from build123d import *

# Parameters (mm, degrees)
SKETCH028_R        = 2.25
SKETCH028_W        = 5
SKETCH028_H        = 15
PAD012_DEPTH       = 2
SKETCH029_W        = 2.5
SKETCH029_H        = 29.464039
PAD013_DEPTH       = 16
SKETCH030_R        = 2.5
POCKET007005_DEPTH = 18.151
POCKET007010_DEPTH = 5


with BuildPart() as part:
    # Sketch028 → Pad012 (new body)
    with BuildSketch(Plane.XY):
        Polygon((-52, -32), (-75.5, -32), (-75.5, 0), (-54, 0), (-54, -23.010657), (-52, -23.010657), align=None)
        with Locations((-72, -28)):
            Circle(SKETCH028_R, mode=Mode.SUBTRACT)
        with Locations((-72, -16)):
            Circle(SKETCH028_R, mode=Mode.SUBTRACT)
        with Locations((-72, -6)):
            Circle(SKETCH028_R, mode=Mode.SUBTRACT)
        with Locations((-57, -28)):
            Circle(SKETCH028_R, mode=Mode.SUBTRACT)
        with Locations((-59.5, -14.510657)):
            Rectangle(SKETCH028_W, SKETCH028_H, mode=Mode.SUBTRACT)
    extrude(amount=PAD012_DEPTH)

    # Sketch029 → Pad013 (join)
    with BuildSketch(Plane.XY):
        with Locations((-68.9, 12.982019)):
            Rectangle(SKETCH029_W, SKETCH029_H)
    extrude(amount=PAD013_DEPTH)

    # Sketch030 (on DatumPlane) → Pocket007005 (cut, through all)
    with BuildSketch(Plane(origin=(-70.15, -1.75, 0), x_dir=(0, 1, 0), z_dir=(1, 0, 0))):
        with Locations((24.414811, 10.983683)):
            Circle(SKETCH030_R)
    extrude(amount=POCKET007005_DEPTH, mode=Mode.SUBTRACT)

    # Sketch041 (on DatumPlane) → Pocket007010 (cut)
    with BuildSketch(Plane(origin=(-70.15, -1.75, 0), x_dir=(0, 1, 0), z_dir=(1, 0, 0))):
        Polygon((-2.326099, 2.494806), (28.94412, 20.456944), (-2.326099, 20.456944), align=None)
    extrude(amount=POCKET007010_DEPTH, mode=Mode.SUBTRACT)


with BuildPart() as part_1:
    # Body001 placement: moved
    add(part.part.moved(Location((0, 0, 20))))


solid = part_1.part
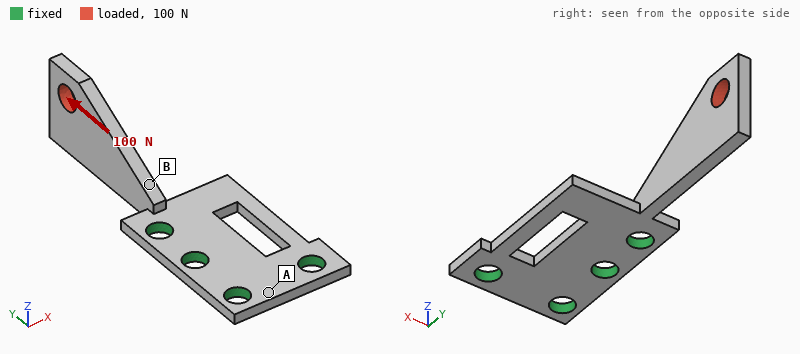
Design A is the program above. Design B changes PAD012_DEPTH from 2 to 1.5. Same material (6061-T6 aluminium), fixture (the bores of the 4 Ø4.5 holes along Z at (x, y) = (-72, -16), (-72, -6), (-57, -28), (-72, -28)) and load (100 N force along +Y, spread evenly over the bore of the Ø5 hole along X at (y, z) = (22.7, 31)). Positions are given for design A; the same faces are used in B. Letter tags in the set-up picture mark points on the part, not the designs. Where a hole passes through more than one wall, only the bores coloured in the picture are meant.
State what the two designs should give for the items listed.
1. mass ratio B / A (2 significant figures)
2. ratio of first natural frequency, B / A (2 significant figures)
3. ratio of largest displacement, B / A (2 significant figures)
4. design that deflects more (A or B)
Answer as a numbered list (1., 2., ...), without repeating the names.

1. 0.85
2. 0.72
3. 1.9
4. B
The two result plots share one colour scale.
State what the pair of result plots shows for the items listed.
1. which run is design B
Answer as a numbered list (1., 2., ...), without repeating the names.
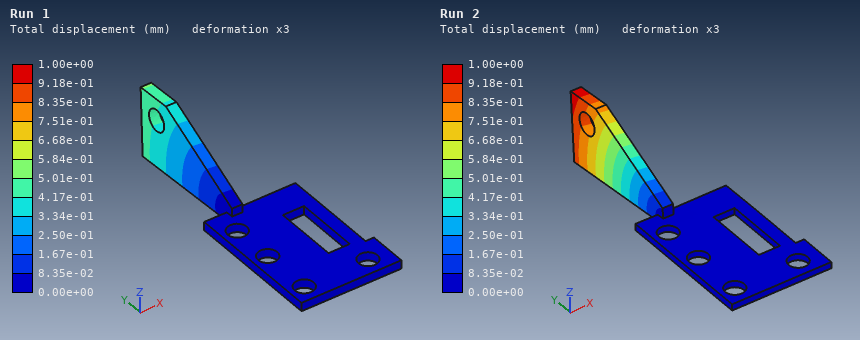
1. Run 2
